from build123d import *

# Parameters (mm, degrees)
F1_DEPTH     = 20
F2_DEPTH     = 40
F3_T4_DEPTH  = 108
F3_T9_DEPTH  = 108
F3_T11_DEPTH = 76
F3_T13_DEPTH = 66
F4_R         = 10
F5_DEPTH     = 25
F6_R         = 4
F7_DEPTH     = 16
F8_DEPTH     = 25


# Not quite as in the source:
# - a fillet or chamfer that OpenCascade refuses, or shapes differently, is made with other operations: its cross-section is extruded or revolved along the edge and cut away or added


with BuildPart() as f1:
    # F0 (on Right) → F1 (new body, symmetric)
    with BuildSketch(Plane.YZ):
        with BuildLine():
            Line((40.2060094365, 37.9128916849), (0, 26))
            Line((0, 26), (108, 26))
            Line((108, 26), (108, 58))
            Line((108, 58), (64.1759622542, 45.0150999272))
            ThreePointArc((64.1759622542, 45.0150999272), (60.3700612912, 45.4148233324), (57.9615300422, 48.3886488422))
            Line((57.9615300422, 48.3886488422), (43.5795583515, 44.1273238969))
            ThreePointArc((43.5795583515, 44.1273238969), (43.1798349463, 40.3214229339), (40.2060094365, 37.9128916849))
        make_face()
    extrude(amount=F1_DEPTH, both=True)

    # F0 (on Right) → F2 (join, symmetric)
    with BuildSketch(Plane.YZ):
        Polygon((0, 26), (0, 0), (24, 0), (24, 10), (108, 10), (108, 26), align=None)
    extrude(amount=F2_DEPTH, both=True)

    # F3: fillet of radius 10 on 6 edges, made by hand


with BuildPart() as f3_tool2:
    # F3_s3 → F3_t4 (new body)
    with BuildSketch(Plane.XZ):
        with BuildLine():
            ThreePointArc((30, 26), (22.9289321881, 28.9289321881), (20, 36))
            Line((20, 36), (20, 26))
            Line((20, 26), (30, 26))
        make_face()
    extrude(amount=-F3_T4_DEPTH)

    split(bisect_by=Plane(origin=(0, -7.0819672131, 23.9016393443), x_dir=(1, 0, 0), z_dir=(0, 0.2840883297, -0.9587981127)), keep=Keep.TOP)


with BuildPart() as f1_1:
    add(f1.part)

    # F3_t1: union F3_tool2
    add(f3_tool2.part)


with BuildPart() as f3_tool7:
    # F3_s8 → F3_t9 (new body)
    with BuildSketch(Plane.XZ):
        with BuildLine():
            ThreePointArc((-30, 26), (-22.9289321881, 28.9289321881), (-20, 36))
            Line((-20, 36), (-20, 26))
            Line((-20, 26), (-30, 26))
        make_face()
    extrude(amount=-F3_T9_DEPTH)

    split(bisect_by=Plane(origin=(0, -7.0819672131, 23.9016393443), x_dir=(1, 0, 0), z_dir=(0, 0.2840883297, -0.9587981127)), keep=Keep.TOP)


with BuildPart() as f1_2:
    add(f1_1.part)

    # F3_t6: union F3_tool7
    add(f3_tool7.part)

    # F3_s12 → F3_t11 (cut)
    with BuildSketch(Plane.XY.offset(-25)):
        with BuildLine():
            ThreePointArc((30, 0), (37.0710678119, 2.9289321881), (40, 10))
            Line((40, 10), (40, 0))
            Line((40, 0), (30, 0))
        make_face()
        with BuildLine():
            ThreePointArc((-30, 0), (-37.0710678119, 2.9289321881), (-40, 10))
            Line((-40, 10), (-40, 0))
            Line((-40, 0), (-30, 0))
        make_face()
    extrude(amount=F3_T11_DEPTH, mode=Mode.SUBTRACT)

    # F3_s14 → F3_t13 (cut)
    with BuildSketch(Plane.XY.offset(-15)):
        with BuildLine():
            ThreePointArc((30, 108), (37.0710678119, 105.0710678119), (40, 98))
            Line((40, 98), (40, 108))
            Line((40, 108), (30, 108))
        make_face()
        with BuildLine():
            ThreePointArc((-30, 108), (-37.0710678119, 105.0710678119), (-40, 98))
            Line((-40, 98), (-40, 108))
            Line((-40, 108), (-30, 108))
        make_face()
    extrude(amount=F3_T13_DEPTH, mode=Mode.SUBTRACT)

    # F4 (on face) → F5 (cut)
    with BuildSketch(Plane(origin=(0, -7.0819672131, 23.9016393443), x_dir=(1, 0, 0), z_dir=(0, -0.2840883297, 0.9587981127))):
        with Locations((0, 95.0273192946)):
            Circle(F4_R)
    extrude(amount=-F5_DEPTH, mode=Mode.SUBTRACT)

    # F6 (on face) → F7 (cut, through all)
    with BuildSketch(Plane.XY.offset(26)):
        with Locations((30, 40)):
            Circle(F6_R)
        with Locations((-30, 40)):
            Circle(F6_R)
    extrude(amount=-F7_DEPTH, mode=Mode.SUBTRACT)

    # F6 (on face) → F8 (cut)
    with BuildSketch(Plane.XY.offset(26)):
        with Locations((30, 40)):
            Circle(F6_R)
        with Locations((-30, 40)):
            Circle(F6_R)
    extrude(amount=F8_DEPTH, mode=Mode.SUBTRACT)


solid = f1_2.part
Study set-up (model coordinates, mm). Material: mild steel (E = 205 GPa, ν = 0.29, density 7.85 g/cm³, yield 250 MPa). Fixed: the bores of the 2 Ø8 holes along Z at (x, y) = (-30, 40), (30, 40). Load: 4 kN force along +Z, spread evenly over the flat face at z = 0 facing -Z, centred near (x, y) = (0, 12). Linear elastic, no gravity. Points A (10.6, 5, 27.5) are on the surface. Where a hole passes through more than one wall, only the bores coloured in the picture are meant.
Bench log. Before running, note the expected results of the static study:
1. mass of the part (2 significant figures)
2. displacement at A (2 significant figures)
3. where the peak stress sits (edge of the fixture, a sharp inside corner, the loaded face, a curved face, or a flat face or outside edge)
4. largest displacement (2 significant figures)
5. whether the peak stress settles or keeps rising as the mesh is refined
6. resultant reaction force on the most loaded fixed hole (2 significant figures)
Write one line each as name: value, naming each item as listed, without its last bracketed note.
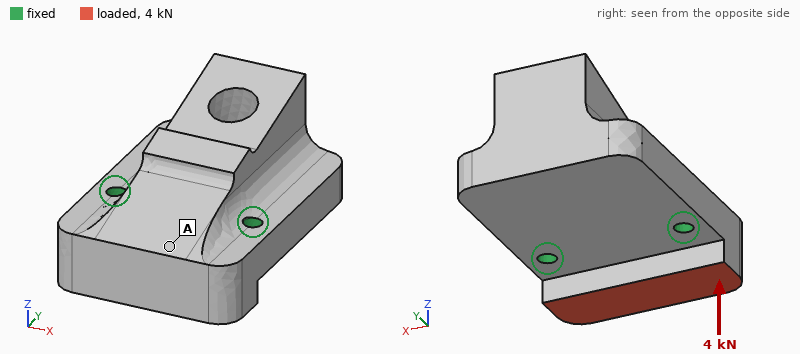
mass of the part: 1.8 kg
displacement at A: 8.6 µm
where the peak stress sits: edge of the fixture
largest displacement: 11 µm
whether the peak stress settles or keeps rising as the mesh is refined: keeps rising
resultant reaction force on the most loaded fixed hole: 2.1 kN
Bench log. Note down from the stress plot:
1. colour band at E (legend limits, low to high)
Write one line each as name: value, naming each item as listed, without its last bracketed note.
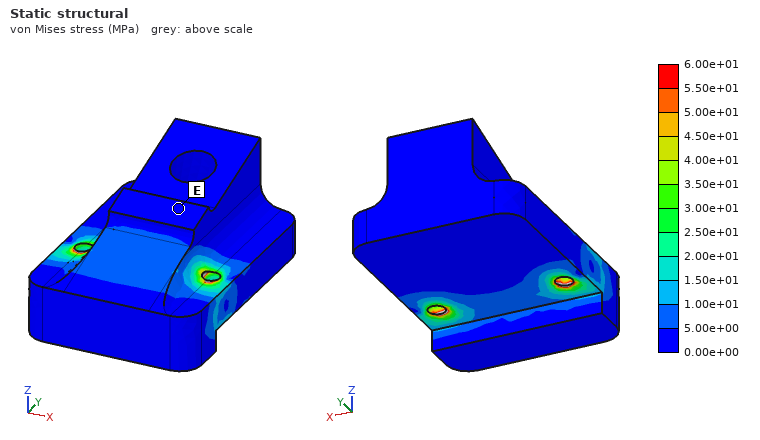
colour band at E: 0.00e+00 to 5.00e+00 MPa
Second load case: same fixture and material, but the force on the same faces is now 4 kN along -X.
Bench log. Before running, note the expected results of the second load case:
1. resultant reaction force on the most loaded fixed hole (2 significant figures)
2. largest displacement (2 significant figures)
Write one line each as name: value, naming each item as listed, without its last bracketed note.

resultant reaction force on the most loaded fixed hole: 2.9 kN
largest displacement: 4.1 µm
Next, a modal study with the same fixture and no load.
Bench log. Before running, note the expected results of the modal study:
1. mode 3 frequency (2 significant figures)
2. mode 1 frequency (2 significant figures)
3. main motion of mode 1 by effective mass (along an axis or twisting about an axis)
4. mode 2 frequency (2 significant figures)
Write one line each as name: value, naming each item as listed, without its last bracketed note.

mode 3 frequency: 6700 Hz
mode 1 frequency: 2300 Hz
main motion of mode 1 by effective mass: along Z
mode 2 frequency: 6600 Hz
